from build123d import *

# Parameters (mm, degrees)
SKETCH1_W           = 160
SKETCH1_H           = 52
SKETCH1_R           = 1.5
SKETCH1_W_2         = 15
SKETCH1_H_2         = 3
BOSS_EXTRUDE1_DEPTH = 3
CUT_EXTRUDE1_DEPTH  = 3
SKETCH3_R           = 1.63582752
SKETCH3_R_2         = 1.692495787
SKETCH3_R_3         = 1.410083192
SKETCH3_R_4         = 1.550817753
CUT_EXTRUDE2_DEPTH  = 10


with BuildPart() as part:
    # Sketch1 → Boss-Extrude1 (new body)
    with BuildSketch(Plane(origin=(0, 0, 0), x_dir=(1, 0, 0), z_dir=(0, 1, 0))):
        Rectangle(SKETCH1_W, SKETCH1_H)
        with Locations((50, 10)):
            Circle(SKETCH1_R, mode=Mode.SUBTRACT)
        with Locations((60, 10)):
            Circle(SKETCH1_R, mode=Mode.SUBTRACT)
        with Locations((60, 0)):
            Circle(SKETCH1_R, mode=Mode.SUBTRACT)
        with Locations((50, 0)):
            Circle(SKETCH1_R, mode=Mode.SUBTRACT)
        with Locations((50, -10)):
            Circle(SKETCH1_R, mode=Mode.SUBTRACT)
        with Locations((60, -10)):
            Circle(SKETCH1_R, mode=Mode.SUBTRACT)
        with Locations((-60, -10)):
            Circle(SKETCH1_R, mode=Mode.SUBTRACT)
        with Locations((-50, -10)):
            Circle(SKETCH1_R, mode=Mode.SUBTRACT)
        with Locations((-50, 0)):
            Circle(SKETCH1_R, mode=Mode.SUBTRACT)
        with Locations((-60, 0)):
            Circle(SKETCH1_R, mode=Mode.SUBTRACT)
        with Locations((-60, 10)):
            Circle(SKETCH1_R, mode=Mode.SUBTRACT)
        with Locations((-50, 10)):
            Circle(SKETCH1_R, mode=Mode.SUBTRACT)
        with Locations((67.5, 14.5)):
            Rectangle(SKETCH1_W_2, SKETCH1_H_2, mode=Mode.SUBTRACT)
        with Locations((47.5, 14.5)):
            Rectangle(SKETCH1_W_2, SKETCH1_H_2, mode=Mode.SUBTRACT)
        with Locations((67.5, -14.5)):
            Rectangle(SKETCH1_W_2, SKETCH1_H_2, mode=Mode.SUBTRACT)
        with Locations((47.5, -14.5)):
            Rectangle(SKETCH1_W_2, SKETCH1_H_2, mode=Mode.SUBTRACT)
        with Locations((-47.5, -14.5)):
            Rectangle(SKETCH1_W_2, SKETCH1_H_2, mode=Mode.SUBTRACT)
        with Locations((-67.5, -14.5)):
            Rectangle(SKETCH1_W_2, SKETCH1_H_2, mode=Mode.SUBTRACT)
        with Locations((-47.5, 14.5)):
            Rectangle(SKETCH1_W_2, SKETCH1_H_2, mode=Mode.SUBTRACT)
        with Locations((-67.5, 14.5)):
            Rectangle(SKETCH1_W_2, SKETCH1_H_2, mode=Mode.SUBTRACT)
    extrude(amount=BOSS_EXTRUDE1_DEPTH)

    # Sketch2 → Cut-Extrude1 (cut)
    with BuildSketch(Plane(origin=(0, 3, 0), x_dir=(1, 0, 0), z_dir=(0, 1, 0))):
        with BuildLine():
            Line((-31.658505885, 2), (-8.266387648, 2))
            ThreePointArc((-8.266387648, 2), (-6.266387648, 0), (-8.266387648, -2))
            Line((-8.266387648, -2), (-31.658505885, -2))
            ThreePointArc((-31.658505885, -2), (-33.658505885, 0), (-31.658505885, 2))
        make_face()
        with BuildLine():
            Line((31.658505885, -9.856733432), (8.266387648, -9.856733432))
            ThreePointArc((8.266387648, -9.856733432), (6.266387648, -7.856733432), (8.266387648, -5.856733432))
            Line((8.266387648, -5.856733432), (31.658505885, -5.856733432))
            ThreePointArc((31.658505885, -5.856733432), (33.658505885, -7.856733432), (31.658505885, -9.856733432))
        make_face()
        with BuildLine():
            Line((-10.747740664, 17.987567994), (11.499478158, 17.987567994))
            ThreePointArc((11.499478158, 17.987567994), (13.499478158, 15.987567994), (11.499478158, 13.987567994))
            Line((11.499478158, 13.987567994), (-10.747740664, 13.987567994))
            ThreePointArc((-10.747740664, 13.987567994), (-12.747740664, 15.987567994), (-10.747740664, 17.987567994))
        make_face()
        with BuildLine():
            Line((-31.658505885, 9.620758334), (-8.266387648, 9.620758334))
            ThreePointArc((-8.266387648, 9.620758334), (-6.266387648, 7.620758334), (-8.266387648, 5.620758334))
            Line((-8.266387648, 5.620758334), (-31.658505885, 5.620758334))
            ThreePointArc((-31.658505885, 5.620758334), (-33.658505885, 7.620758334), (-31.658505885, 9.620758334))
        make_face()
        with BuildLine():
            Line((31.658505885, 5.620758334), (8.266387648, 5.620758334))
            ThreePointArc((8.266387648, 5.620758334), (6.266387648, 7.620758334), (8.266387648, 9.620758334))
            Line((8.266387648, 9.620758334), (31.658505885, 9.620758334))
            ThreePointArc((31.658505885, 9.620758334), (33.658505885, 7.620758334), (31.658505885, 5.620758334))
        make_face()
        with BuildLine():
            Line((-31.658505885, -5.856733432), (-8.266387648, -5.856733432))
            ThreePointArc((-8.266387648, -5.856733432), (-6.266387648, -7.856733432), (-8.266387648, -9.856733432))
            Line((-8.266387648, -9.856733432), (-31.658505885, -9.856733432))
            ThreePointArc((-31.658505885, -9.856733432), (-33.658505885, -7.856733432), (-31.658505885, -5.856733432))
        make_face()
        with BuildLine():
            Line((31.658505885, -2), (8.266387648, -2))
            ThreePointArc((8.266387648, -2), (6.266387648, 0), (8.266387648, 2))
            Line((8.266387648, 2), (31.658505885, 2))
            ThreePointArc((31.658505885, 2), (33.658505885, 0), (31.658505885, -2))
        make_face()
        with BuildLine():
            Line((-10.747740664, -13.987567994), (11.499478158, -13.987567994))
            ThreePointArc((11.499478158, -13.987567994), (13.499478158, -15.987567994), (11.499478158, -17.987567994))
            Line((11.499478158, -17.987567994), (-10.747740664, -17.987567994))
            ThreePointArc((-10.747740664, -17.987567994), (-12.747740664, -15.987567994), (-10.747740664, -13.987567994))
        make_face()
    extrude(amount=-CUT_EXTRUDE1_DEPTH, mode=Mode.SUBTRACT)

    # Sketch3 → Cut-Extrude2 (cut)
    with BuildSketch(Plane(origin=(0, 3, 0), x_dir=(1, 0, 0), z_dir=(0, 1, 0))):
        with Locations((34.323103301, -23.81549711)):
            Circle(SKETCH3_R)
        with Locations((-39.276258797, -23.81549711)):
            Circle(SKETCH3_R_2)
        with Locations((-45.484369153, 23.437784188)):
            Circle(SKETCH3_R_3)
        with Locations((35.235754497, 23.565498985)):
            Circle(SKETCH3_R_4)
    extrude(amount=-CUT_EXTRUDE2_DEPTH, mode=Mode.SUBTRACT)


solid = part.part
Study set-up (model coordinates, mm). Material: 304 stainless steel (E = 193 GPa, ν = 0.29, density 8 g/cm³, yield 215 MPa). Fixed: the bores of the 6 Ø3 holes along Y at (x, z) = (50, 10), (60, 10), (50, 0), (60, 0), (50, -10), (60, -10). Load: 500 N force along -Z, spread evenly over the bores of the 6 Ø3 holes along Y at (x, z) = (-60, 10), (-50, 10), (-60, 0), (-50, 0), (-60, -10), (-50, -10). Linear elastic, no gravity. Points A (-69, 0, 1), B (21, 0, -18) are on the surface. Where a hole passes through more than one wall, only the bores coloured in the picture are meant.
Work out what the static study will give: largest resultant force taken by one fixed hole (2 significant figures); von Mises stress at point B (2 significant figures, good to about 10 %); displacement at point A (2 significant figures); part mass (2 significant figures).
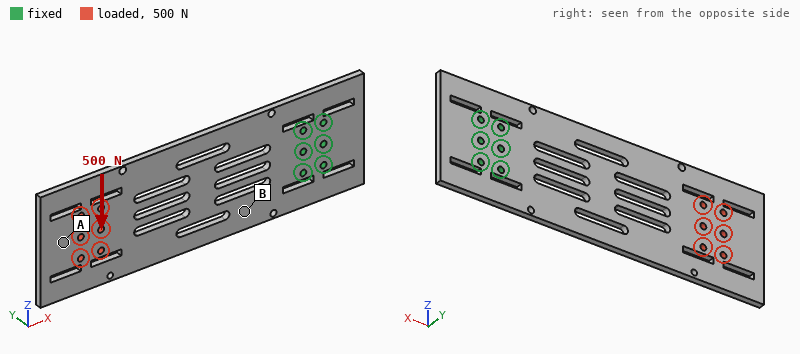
1.2 kN
22 MPa
0.11 mm
170 g
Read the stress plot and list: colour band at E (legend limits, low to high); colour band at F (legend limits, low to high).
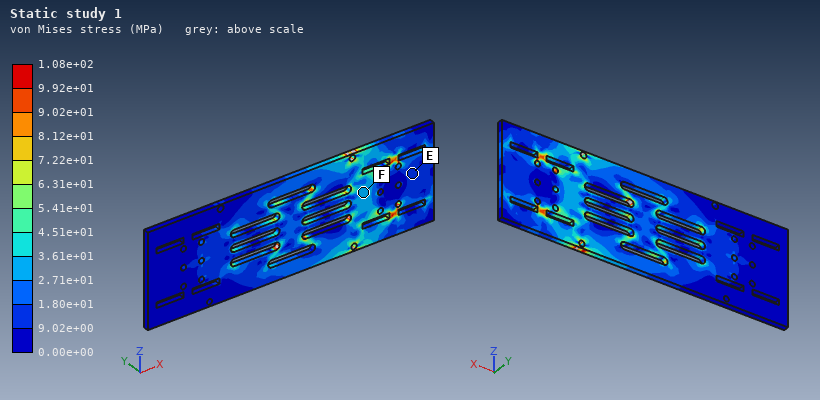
9.02e+00 to 1.80e+01 MPa
2.71e+01 to 3.61e+01 MPa
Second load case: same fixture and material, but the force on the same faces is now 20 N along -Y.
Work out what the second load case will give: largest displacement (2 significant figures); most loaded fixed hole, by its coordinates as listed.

0.61 mm
(50, 0)
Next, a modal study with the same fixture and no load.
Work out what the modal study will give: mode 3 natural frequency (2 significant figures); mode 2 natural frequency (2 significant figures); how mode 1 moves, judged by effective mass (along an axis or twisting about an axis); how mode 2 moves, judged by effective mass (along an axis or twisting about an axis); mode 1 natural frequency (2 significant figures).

850 Hz
590 Hz
along Y
twisting about X
130 Hz
